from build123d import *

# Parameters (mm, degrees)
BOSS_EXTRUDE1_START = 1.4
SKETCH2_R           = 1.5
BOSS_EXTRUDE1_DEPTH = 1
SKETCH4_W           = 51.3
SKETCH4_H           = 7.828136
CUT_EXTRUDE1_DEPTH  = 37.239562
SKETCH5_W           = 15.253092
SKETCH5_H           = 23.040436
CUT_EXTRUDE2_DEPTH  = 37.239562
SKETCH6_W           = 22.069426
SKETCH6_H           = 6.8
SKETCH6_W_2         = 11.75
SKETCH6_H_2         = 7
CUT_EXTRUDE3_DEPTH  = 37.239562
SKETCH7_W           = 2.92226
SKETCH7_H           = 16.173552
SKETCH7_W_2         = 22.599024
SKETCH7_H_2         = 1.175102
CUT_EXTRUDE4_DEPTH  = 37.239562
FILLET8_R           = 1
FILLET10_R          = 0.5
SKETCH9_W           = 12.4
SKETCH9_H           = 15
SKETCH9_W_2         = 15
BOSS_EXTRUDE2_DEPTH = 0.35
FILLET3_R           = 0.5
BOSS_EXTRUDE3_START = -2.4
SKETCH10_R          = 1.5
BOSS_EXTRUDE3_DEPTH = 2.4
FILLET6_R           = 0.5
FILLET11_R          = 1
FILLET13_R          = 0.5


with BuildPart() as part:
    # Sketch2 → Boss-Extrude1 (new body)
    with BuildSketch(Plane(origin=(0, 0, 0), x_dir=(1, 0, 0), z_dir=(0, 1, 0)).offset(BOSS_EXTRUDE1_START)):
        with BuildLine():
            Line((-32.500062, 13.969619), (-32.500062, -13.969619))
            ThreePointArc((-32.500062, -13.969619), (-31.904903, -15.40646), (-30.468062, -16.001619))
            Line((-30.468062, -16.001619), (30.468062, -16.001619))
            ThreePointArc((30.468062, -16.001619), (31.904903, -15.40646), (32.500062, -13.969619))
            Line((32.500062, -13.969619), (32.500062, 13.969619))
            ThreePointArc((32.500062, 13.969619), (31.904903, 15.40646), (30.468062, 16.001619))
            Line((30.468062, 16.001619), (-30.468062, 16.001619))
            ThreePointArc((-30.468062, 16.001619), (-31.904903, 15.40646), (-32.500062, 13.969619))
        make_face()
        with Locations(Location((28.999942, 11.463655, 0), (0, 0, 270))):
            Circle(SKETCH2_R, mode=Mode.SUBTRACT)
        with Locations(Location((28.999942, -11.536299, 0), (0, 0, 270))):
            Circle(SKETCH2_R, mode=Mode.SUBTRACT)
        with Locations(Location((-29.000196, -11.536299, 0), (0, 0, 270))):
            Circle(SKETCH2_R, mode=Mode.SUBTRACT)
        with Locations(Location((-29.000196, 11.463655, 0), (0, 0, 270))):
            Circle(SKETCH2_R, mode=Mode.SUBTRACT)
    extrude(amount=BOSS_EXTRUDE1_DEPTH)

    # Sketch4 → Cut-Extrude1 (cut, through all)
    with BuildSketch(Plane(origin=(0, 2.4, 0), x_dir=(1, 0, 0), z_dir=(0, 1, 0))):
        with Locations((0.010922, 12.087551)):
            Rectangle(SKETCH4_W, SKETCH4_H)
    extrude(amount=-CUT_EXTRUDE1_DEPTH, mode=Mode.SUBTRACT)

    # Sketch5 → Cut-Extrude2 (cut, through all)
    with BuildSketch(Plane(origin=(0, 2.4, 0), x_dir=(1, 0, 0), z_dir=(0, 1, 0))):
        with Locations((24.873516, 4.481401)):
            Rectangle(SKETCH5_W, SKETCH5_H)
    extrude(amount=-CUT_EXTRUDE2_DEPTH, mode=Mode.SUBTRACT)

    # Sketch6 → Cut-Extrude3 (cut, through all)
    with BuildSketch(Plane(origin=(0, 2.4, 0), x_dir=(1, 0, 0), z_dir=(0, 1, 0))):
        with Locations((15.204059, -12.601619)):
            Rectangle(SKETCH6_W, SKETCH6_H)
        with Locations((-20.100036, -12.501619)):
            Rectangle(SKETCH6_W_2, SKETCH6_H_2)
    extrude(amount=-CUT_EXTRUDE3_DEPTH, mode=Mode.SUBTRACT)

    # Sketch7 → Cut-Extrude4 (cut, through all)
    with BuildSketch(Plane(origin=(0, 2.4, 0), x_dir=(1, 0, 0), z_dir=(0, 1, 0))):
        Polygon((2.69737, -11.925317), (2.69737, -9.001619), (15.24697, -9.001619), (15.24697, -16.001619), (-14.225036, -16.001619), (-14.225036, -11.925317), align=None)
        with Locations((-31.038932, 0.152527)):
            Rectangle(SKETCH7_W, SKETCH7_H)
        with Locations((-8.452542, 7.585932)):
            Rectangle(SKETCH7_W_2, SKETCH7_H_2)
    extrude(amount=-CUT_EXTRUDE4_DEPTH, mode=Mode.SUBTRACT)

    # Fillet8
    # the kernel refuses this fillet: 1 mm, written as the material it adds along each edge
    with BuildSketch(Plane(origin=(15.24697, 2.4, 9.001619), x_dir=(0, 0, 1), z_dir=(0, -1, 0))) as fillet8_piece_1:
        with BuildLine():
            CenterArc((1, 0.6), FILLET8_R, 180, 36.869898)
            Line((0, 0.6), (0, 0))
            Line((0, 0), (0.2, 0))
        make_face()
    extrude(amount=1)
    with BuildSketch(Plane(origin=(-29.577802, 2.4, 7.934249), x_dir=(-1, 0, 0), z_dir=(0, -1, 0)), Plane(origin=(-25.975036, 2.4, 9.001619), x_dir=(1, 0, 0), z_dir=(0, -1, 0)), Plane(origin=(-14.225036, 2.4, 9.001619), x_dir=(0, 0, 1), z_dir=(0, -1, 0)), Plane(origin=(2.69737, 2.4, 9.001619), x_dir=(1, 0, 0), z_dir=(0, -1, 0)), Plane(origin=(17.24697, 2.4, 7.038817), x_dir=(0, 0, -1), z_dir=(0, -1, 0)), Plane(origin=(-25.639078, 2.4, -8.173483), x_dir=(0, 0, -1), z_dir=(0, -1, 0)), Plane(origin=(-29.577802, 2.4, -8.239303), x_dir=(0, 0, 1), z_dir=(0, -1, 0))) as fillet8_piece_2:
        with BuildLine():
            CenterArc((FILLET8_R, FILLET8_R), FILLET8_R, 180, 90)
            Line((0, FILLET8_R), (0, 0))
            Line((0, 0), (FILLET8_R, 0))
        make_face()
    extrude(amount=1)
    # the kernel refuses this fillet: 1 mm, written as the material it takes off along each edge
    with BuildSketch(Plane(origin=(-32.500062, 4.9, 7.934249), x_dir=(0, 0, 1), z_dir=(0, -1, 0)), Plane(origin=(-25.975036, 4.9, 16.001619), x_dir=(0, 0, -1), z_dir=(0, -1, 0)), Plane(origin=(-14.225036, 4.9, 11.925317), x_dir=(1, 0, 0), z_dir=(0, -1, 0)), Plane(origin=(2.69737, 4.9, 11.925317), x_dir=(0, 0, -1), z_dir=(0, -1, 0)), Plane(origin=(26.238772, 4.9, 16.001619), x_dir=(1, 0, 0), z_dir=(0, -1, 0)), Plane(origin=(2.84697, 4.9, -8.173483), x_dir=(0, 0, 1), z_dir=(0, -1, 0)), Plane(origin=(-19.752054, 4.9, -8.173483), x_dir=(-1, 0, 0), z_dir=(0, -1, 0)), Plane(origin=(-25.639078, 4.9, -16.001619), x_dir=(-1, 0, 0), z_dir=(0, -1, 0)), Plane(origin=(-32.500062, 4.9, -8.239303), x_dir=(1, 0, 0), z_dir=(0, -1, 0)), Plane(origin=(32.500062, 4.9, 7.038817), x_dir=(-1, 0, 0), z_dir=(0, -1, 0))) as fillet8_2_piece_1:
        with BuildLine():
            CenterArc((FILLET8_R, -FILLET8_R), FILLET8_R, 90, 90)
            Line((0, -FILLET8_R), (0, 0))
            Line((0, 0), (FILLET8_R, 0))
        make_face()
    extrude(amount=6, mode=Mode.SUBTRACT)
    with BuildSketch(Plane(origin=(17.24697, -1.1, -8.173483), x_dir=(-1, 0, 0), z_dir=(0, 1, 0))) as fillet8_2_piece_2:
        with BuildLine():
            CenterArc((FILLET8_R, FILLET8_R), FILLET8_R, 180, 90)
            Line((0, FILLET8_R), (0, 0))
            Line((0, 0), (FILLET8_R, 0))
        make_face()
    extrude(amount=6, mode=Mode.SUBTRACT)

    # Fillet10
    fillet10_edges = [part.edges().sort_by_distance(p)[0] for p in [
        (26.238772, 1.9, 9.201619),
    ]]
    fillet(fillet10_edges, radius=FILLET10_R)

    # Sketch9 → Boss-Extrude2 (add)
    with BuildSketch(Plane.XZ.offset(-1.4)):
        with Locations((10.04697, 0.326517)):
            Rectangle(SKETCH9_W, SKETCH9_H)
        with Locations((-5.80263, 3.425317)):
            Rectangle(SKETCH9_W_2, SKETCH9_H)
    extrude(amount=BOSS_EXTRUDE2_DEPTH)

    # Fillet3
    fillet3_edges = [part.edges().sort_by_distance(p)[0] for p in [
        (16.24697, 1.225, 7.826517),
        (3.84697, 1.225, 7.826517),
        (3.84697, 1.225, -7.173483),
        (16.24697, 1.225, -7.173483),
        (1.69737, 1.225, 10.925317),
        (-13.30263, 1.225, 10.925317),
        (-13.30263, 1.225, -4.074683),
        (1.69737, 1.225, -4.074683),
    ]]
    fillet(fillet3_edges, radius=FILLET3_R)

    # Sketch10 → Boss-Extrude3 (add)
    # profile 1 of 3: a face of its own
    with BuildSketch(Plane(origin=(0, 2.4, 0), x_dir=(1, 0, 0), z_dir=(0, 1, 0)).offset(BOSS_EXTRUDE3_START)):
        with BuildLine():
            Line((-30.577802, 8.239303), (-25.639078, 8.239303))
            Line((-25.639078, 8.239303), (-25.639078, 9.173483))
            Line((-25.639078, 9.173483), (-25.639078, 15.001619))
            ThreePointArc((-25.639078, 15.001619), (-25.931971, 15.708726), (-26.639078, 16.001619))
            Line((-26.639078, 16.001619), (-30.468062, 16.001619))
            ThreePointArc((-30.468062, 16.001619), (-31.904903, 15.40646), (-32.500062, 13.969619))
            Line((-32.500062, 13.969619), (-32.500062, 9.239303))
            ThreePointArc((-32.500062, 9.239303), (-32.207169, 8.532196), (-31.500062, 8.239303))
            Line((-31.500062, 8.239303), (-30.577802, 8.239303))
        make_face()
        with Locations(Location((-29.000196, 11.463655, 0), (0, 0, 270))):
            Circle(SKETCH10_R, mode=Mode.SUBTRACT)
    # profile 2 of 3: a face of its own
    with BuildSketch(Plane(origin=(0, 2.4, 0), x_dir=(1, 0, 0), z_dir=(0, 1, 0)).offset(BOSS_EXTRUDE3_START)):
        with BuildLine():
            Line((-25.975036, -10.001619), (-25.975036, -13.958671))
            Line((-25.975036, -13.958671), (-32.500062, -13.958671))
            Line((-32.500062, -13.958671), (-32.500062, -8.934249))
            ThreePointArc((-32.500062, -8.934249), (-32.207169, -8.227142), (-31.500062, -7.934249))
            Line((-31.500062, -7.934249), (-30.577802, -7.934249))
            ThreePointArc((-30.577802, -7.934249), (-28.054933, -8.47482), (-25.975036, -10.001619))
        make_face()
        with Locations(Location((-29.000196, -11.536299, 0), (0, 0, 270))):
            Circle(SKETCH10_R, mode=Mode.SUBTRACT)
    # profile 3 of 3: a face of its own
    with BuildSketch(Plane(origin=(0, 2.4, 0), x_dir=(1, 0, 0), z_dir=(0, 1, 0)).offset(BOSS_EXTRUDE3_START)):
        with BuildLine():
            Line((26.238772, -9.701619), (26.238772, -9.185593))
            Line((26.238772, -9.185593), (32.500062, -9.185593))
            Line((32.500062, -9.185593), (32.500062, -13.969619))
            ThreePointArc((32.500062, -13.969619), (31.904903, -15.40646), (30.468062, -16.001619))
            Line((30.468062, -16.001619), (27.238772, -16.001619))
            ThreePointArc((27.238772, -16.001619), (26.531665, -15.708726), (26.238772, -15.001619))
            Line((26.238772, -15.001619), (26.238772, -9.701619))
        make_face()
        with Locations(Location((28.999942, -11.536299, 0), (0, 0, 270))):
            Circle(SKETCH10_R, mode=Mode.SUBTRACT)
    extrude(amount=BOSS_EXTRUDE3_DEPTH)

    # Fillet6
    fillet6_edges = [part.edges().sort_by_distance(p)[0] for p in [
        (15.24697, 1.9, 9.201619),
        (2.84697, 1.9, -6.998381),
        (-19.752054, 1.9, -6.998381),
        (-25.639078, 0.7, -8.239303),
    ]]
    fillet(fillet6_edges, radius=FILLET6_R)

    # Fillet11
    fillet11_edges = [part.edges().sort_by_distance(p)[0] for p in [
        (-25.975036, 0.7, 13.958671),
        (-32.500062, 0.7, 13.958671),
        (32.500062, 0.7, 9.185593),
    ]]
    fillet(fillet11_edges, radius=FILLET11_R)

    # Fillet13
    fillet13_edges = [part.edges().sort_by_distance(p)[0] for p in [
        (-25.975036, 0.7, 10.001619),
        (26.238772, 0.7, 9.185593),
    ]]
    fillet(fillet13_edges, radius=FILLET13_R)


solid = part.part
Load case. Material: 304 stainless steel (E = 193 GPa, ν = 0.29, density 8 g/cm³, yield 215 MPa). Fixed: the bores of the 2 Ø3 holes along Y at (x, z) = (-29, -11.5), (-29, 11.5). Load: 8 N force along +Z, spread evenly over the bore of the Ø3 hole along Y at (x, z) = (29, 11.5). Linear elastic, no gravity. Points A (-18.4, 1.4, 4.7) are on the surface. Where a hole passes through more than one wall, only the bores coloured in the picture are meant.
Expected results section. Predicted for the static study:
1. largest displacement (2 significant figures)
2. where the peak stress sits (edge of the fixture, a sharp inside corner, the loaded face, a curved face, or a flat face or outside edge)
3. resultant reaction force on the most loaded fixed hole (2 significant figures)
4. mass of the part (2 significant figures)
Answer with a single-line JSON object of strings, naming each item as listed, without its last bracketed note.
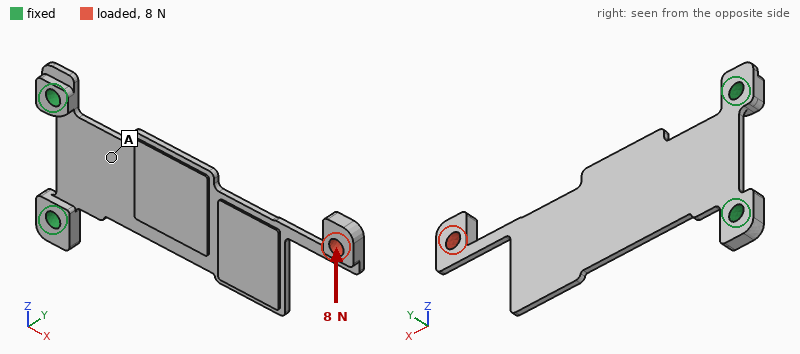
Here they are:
{"largest displacement": "66 µm", "where the peak stress sits": "a curved face", "resultant reaction force on the most loaded fixed hole": "26 N", "mass of the part": "10 g"}
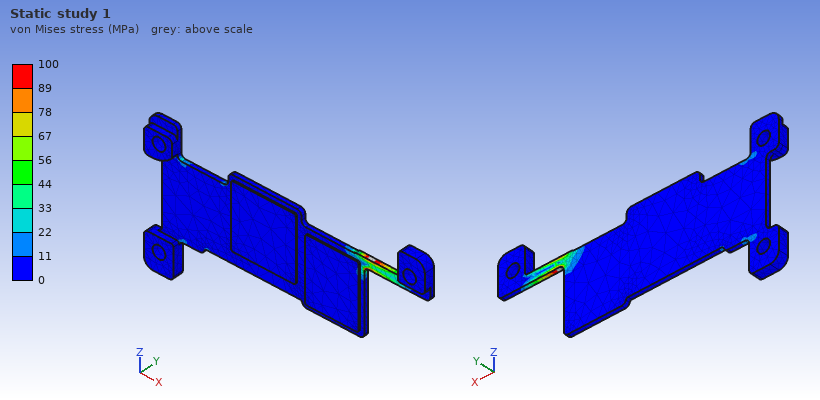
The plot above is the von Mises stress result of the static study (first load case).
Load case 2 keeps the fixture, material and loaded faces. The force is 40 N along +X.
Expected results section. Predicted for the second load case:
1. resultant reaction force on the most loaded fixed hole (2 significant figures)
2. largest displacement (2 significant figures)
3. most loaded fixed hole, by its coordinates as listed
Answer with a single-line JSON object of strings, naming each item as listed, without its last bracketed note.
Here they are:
{"resultant reaction force on the most loaded fixed hole": "47 N", "largest displacement": "0.27 mm", "most loaded fixed hole, by its coordinates as listed": "(-29, 11.5)"}
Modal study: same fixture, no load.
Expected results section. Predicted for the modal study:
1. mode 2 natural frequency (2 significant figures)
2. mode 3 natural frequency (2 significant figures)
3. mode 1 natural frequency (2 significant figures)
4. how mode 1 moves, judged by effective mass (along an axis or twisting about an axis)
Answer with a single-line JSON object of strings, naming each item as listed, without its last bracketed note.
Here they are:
{"mode 2 natural frequency": "990 Hz", "mode 3 natural frequency": "2000 Hz", "mode 1 natural frequency": "250 Hz", "how mode 1 moves, judged by effective mass": "along Y"}
